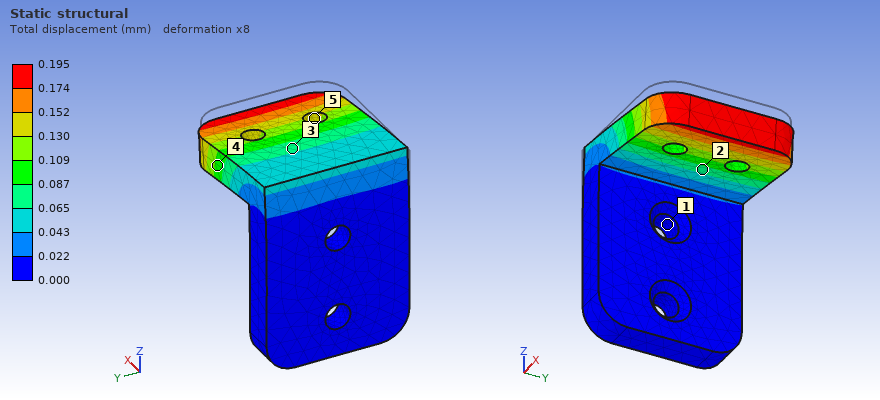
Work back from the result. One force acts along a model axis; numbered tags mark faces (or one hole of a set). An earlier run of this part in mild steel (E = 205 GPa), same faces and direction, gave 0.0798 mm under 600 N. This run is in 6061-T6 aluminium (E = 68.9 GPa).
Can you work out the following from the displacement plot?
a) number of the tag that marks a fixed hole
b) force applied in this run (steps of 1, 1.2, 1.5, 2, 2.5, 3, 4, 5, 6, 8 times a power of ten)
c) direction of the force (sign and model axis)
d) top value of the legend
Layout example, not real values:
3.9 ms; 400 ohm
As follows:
1; 500 N; -Z; 0.195 mm
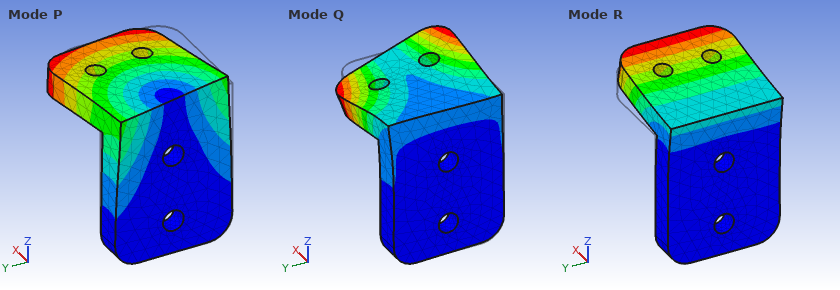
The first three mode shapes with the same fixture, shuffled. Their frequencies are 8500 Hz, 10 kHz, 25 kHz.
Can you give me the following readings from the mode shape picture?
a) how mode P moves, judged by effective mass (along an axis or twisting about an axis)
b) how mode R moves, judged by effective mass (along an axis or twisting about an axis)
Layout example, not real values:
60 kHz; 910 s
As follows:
along Y; along Z
